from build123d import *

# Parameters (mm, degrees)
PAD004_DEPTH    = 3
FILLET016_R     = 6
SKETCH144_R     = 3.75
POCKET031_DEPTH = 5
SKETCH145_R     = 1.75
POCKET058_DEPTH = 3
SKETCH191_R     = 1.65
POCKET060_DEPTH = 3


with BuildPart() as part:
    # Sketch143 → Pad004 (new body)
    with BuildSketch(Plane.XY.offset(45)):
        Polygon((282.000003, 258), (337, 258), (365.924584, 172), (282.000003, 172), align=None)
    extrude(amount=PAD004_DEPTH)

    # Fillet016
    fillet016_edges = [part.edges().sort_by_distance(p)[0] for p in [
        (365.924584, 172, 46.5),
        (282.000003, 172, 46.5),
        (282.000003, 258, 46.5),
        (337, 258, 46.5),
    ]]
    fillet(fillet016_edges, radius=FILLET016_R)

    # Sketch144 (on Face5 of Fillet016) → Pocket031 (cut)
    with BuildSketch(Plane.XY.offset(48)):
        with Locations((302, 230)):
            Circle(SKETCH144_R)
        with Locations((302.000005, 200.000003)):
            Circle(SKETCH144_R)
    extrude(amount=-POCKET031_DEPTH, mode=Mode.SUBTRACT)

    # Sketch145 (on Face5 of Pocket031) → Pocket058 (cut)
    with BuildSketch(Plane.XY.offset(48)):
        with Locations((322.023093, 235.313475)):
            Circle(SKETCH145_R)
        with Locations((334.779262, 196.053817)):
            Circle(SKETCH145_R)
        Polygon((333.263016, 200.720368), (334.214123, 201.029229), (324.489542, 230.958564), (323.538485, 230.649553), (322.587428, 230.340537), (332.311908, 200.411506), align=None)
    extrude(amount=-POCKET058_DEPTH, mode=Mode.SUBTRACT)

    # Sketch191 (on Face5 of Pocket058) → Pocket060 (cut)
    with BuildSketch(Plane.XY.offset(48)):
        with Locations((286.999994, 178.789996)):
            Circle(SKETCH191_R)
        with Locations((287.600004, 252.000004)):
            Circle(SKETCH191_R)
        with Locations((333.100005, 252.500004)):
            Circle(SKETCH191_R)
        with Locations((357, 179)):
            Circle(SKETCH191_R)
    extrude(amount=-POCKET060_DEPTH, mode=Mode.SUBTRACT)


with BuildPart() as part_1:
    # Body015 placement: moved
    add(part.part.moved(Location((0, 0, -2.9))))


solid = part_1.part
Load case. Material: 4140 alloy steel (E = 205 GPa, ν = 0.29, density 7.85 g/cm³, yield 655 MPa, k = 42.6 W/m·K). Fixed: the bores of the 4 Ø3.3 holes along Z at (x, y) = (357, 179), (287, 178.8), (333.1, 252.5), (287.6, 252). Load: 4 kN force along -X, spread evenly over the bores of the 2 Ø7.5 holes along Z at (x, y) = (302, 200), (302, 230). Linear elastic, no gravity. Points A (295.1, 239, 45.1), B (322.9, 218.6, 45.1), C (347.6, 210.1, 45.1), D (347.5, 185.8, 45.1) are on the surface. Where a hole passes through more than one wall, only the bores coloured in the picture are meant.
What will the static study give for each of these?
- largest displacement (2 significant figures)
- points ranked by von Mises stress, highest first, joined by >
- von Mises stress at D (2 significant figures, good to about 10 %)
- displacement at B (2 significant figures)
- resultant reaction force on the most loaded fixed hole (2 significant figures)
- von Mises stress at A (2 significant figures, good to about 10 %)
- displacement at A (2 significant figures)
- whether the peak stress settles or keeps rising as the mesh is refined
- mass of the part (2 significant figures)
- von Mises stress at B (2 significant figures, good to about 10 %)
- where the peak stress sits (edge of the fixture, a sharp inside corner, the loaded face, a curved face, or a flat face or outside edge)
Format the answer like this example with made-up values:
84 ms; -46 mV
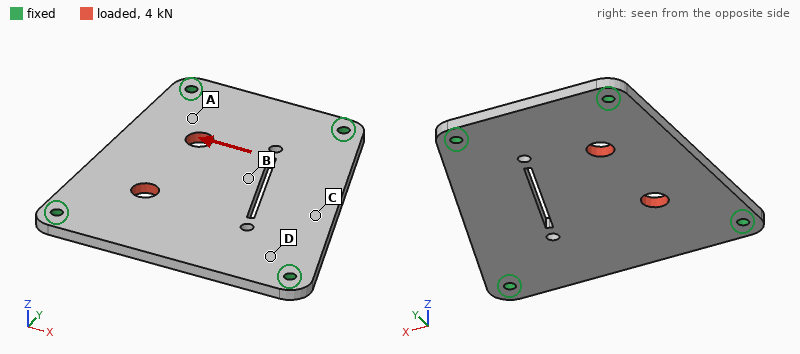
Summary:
6.9 µm; A > D > B > C; 18 MPa; 5.6 µm; 1.3 kN; 25 MPa; 3.5 µm; keeps rising; 140 g; 11 MPa; edge of the fixture
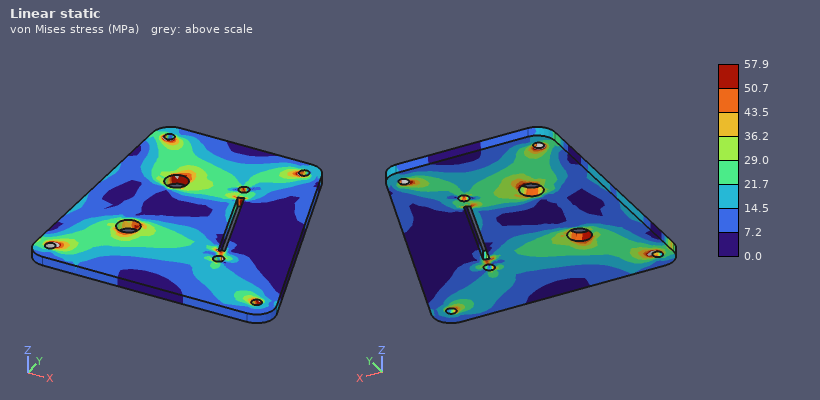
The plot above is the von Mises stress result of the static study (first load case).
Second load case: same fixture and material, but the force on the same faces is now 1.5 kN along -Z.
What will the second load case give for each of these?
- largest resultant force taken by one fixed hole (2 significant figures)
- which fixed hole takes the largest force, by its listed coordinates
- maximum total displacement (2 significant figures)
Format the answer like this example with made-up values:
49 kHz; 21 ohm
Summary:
620 N; (287, 178.8); 0.15 mm
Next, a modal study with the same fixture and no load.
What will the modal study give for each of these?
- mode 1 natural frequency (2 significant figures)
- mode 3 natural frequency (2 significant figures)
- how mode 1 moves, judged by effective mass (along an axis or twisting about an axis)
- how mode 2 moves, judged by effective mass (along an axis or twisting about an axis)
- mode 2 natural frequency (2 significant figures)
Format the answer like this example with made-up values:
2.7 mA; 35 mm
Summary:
2100 Hz; 3600 Hz; along Z; twisting about Y; 3200 Hz
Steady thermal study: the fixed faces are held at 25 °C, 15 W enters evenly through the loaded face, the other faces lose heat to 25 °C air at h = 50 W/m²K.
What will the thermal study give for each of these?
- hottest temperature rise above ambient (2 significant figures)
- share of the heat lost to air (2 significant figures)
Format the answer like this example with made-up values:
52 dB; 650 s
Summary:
34 K; 50 %
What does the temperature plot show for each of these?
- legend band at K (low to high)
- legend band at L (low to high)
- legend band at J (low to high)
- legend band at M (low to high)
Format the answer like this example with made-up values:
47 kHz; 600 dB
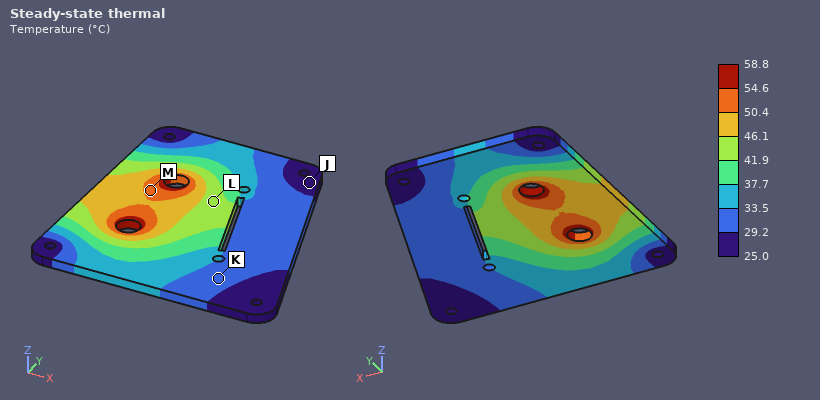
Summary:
29.2 to 33.5 °C; 41.9 to 46.1 °C; 25.0 to 29.2 °C; 50.4 to 54.6 °C
